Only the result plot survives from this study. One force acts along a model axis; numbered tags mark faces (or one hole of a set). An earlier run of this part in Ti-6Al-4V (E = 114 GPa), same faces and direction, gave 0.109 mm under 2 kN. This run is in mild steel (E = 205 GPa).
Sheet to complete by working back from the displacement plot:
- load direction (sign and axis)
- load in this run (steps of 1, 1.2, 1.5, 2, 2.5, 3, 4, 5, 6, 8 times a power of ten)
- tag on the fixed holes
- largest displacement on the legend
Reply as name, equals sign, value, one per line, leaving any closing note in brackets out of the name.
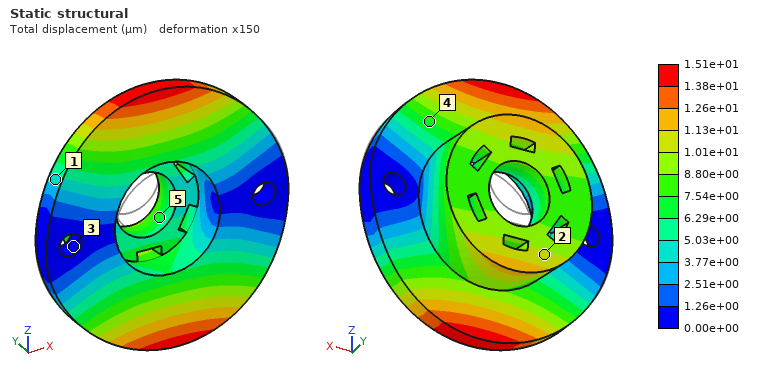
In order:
load direction = -Z
load in this run = 500 N
tag on the fixed holes = 3
largest displacement on the legend = 1.51e+01 µm
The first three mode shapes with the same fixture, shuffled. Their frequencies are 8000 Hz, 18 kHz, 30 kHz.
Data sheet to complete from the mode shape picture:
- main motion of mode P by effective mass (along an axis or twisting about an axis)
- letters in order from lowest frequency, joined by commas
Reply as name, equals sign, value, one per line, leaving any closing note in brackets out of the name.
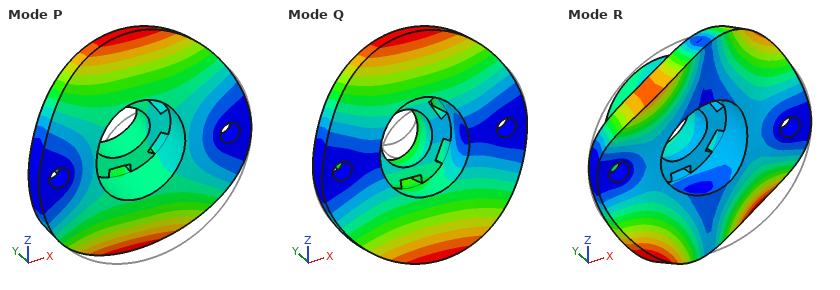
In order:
main motion of mode P by effective mass = along Y
letters in order from lowest frequency, joined by commas = Q, P, R
